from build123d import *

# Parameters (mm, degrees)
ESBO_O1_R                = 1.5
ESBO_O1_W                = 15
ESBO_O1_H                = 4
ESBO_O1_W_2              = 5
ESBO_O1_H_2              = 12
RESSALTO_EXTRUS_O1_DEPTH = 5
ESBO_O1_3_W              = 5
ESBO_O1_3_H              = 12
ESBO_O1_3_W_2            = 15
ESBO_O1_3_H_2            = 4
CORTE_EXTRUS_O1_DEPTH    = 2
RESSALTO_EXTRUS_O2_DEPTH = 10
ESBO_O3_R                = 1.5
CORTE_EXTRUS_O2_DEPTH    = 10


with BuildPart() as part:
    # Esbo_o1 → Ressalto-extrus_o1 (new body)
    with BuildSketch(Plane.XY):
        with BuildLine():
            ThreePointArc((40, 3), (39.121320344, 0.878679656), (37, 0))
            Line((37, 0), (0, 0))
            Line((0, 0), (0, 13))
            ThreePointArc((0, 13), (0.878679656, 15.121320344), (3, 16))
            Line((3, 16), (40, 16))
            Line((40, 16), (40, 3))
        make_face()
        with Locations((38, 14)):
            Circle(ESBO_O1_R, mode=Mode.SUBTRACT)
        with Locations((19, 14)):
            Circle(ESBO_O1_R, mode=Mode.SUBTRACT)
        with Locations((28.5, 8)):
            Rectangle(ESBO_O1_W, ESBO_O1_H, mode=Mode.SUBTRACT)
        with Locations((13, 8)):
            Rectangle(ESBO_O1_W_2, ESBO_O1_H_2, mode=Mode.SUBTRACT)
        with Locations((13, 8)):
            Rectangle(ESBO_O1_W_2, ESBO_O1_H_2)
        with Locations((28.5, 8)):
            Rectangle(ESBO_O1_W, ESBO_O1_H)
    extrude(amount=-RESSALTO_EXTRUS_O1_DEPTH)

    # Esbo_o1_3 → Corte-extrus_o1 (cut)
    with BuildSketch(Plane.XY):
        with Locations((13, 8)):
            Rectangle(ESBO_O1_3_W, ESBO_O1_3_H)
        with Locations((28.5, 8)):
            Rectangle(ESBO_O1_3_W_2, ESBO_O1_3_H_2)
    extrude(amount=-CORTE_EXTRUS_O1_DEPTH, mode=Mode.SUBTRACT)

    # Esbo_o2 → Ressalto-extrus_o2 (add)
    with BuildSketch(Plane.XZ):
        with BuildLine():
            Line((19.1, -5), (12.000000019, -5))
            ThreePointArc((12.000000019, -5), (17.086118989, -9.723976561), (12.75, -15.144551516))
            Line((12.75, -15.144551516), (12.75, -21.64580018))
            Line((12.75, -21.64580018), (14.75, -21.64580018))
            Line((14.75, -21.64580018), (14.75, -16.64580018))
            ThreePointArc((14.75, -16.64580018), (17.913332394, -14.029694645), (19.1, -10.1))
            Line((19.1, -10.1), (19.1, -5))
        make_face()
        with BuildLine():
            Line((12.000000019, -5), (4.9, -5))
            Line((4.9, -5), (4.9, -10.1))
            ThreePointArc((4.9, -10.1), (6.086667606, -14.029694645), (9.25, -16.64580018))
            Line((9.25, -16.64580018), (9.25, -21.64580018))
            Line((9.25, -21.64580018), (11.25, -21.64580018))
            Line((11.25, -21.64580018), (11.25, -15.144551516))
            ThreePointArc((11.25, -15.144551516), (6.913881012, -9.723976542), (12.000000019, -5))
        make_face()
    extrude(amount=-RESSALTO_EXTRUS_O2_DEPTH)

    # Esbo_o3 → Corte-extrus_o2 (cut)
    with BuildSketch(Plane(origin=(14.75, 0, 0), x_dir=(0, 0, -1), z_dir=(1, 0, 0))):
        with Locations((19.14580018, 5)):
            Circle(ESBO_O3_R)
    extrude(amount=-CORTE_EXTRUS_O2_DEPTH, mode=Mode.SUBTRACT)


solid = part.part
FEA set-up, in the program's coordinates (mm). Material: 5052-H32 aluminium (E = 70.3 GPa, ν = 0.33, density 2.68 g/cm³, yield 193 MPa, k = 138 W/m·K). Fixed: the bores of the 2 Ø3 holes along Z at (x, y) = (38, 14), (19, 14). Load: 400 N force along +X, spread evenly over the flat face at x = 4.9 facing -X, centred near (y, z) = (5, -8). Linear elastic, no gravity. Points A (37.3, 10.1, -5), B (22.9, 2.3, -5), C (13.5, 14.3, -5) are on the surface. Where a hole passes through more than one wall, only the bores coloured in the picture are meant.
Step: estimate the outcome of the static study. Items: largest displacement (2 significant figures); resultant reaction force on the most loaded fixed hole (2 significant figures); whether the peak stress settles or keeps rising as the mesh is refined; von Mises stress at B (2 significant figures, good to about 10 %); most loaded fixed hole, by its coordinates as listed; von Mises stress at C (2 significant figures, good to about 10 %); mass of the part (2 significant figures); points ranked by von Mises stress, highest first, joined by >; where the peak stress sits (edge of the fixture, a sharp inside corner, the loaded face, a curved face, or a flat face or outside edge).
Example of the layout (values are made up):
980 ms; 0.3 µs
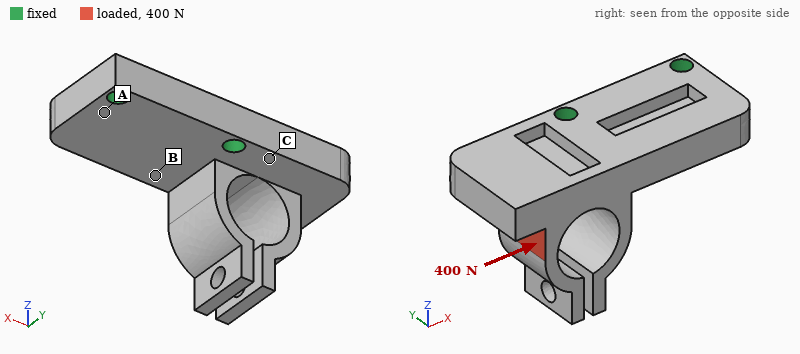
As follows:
79 µm; 270 N; keeps rising; 22 MPa; (19, 14); 40 MPa; 9.9 g; C > B > A; edge of the fixture
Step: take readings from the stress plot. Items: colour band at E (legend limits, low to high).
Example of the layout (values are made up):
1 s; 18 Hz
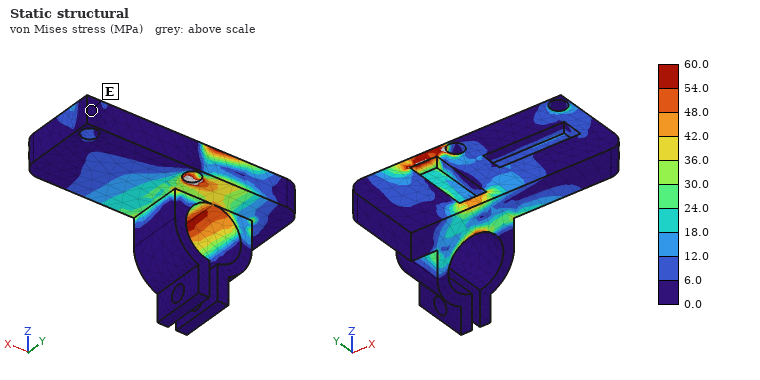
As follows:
0.0 to 6.0 MPa
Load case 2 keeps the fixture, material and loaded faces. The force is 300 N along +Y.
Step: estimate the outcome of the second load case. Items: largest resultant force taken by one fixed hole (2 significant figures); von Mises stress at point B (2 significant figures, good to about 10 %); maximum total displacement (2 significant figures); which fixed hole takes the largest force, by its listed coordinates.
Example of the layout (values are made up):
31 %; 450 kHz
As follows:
500 N; 9.5 MPa; 44 µm; (19, 14)
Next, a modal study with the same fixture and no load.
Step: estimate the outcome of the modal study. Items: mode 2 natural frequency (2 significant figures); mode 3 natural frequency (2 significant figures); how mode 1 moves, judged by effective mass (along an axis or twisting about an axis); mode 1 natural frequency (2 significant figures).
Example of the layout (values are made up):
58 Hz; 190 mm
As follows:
6600 Hz; 7400 Hz; along Z; 5100 Hz
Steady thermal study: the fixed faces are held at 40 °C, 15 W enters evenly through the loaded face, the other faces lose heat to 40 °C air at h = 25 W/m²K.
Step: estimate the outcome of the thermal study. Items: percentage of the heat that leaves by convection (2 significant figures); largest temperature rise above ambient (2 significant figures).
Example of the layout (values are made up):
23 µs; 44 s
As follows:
6.0 %; 37 K
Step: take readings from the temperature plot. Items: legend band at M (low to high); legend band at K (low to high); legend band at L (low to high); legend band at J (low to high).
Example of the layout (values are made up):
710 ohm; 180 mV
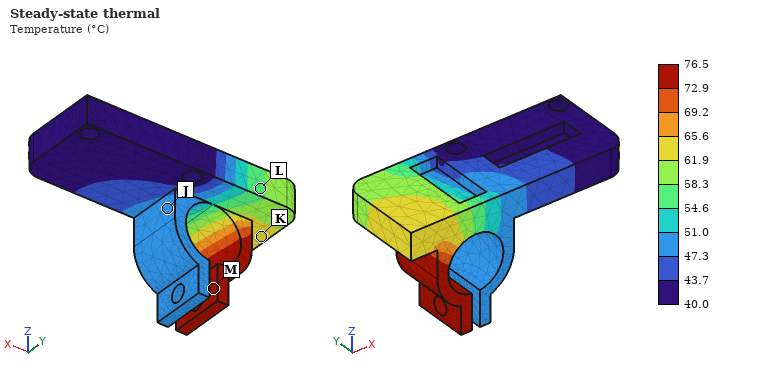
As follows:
72.9 to 76.5 °C; 61.9 to 65.6 °C; 54.6 to 58.3 °C; 47.3 to 51.0 °C
